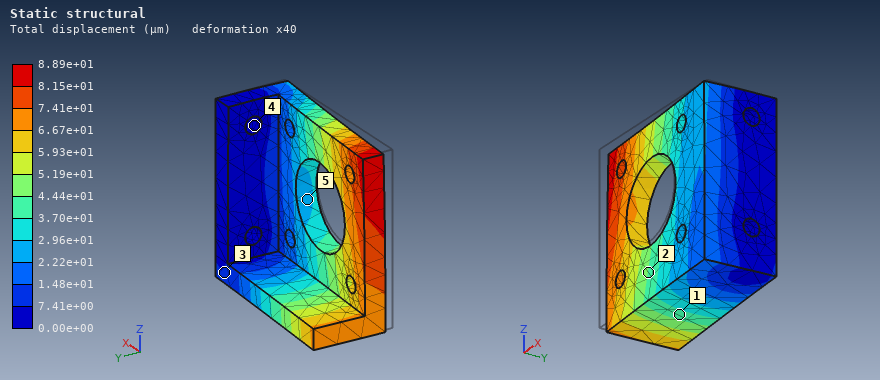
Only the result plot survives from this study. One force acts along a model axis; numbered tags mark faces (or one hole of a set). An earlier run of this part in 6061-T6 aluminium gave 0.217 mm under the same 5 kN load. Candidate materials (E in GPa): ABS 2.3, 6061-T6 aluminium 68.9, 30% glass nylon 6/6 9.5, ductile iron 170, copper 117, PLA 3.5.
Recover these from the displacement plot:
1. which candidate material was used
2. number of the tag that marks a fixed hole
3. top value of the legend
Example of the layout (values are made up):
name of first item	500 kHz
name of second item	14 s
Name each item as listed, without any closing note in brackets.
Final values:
which candidate material was used	ductile iron
number of the tag that marks a fixed hole	4
top value of the legend	8.89e+01 µm
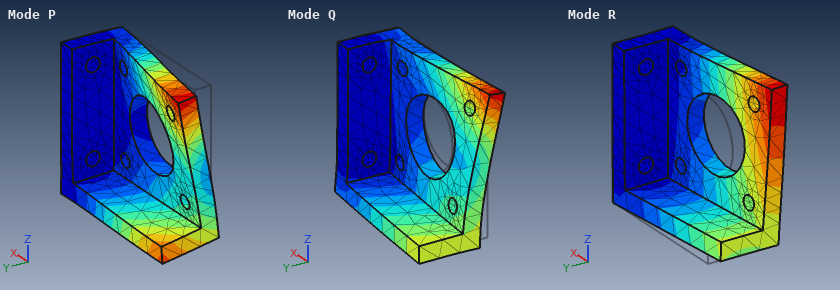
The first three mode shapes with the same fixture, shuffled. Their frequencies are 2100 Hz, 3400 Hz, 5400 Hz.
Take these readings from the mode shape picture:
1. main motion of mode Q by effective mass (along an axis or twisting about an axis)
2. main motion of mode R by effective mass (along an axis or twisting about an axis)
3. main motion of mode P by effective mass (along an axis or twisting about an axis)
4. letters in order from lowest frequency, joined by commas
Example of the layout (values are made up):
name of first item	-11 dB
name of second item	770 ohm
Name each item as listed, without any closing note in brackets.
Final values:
main motion of mode Q by effective mass	along Z
main motion of mode R by effective mass	along Y
main motion of mode P by effective mass	along Z
letters in order from lowest frequency, joined by commas	R, P, Q
